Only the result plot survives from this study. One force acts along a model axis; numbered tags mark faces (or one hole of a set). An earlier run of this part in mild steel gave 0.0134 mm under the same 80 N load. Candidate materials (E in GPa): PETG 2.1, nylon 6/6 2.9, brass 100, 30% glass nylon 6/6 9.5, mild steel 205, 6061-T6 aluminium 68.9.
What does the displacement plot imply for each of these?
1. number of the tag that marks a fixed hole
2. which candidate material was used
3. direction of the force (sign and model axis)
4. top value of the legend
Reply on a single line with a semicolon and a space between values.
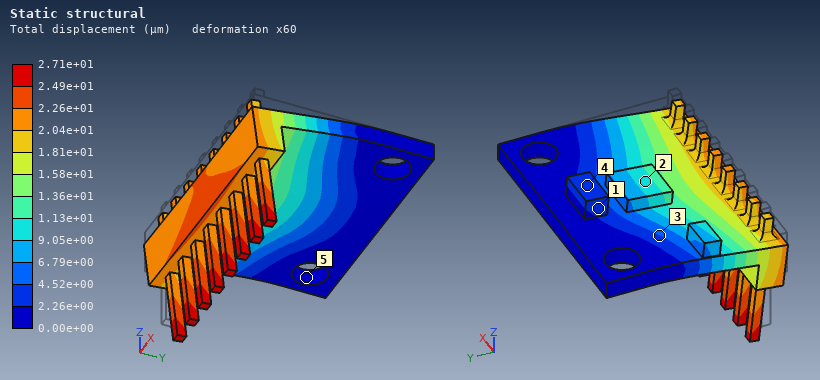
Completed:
5; brass; -Z; 2.71e+01 µm
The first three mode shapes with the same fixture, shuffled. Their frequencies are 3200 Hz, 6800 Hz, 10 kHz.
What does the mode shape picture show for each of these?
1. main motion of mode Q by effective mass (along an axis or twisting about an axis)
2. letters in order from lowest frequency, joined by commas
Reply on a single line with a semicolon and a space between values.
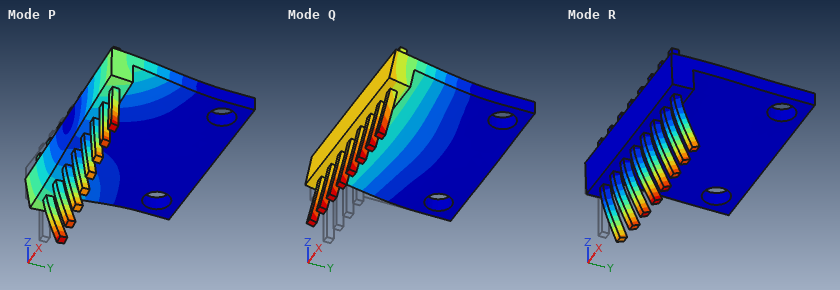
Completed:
along Z; Q, P, R
